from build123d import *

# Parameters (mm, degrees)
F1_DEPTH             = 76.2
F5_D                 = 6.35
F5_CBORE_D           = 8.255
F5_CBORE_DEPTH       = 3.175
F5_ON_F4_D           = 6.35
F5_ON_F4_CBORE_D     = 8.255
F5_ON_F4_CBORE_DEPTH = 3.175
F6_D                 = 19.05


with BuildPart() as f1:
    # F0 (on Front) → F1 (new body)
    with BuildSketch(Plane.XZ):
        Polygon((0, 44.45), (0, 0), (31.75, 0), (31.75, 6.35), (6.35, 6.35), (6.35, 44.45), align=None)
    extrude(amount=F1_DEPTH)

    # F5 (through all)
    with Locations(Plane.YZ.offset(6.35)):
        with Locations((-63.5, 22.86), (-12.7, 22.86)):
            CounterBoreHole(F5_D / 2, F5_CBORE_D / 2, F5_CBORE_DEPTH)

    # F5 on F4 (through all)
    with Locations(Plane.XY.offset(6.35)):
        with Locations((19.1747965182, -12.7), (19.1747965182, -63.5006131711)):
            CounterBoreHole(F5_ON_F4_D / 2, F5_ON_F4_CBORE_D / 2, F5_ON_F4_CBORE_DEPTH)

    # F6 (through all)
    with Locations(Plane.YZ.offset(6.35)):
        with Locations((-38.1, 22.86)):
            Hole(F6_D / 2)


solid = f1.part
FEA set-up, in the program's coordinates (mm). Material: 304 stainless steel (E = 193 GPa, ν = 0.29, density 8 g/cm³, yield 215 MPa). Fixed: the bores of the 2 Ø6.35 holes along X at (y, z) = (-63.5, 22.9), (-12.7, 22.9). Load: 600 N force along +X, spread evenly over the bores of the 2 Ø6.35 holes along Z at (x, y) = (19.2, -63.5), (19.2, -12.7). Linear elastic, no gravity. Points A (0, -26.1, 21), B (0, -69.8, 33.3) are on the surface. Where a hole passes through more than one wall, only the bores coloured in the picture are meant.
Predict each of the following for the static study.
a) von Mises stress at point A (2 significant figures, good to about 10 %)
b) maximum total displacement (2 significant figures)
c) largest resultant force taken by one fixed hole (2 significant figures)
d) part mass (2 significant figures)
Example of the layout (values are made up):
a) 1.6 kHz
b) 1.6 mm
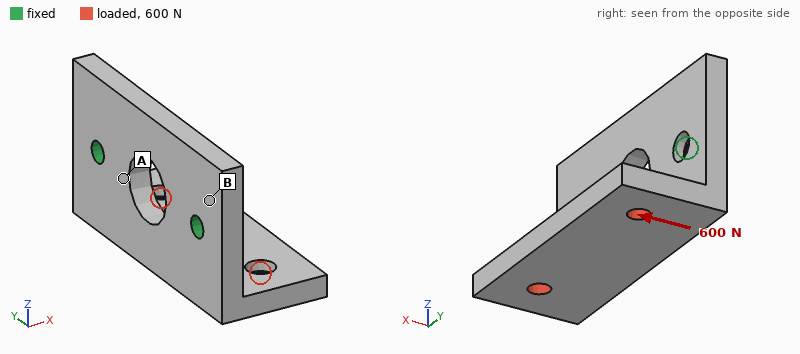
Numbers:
a) 16 MPa
b) 32 µm
c) 300 N
d) 250 g
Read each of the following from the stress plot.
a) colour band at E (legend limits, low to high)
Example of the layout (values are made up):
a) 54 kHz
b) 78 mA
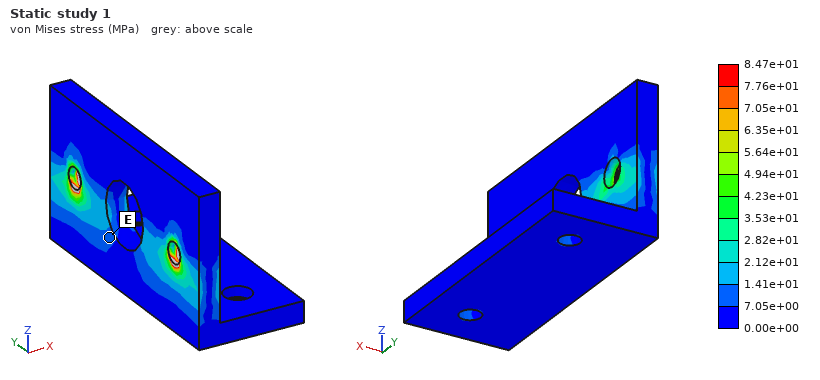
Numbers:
a) 7.05e+00 to 1.41e+01 MPa
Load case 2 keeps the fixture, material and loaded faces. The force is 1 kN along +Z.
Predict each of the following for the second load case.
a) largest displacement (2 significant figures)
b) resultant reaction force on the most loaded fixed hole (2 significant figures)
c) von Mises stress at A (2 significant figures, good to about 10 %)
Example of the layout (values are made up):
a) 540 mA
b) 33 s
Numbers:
a) 64 µm
b) 500 N
c) 28 MPa
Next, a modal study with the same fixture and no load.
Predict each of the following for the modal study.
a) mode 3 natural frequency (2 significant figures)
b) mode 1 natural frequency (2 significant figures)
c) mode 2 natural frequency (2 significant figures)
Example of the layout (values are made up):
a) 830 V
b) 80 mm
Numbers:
a) 6000 Hz
b) 2000 Hz
c) 4000 Hz
